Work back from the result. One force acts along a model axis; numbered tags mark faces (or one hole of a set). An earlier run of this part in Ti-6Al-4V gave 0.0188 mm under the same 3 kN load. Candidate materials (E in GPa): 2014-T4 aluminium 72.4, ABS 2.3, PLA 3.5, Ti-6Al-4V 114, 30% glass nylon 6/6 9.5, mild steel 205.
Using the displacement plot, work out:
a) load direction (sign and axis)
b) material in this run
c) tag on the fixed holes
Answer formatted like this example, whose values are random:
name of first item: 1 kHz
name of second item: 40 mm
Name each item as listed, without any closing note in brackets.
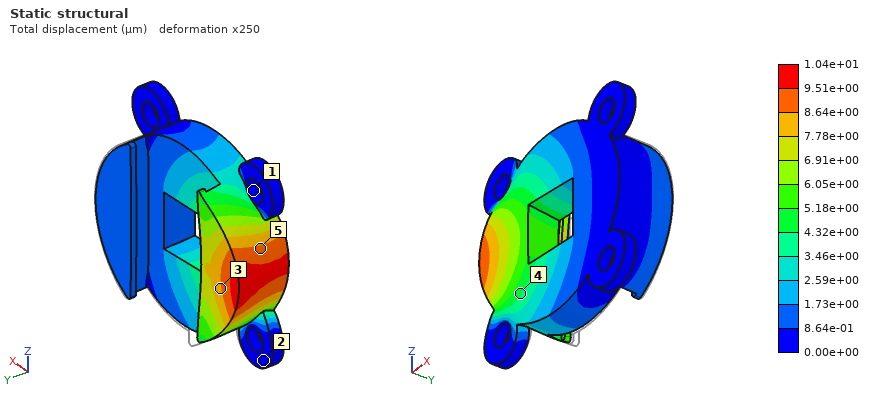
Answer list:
load direction: -Y
material in this run: mild steel
tag on the fixed holes: 1
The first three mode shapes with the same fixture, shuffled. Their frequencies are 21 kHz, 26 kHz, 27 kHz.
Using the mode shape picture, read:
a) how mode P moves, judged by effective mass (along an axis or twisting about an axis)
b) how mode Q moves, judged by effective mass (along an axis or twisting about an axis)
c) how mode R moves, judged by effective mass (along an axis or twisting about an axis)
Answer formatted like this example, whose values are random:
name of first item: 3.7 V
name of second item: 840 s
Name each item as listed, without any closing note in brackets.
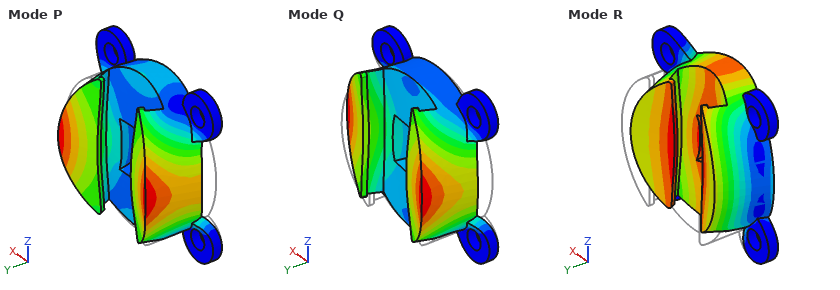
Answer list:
how mode P moves, judged by effective mass: along Y
how mode Q moves, judged by effective mass: along X
how mode R moves, judged by effective mass: along Y
